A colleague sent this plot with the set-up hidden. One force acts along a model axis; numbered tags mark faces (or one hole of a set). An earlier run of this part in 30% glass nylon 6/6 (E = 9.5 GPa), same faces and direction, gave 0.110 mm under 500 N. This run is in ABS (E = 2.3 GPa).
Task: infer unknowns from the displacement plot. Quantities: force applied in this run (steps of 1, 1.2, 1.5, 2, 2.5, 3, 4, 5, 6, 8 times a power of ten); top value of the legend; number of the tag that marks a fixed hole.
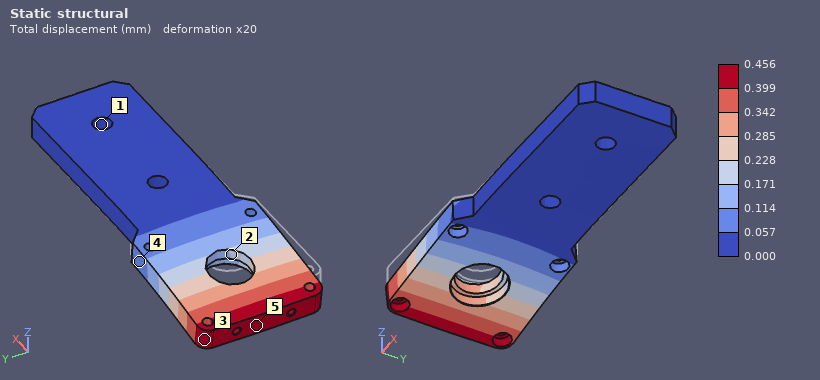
500 N
0.456 mm
1
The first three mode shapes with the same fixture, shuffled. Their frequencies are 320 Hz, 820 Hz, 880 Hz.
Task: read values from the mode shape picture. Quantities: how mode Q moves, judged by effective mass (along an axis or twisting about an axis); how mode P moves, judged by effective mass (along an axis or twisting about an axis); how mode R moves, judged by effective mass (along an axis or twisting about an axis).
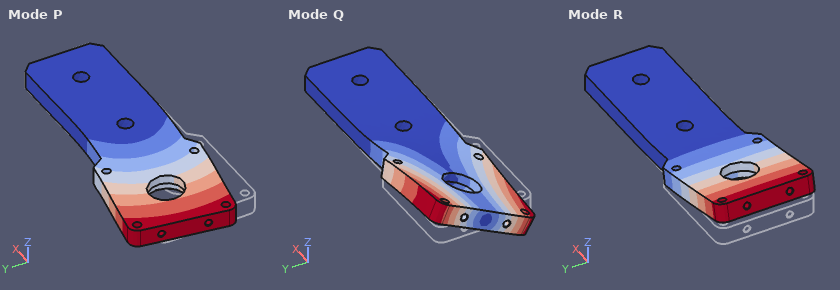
twisting about X
along Y
along Z
